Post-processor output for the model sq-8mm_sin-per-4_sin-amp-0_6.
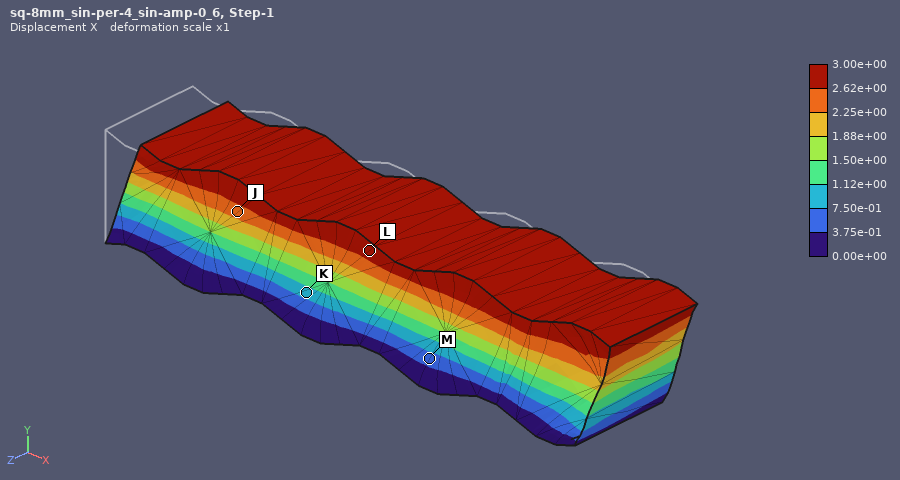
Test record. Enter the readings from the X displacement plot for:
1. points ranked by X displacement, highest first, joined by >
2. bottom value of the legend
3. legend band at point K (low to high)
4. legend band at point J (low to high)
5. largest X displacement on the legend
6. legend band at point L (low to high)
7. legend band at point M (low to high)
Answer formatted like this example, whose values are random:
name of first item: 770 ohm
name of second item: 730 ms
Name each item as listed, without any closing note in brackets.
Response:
points ranked by X displacement, highest first, joined by >: L > J > K > M
bottom value of the legend: 0.00e+00
legend band at point K: 7.50e-01 to 1.12e+00
legend band at point J: 2.25e+00 to 2.62e+00
largest X displacement on the legend: 3.00e+00
legend band at point L: 2.62e+00 to 3.00e+00
legend band at point M: 3.75e-01 to 7.50e-01
